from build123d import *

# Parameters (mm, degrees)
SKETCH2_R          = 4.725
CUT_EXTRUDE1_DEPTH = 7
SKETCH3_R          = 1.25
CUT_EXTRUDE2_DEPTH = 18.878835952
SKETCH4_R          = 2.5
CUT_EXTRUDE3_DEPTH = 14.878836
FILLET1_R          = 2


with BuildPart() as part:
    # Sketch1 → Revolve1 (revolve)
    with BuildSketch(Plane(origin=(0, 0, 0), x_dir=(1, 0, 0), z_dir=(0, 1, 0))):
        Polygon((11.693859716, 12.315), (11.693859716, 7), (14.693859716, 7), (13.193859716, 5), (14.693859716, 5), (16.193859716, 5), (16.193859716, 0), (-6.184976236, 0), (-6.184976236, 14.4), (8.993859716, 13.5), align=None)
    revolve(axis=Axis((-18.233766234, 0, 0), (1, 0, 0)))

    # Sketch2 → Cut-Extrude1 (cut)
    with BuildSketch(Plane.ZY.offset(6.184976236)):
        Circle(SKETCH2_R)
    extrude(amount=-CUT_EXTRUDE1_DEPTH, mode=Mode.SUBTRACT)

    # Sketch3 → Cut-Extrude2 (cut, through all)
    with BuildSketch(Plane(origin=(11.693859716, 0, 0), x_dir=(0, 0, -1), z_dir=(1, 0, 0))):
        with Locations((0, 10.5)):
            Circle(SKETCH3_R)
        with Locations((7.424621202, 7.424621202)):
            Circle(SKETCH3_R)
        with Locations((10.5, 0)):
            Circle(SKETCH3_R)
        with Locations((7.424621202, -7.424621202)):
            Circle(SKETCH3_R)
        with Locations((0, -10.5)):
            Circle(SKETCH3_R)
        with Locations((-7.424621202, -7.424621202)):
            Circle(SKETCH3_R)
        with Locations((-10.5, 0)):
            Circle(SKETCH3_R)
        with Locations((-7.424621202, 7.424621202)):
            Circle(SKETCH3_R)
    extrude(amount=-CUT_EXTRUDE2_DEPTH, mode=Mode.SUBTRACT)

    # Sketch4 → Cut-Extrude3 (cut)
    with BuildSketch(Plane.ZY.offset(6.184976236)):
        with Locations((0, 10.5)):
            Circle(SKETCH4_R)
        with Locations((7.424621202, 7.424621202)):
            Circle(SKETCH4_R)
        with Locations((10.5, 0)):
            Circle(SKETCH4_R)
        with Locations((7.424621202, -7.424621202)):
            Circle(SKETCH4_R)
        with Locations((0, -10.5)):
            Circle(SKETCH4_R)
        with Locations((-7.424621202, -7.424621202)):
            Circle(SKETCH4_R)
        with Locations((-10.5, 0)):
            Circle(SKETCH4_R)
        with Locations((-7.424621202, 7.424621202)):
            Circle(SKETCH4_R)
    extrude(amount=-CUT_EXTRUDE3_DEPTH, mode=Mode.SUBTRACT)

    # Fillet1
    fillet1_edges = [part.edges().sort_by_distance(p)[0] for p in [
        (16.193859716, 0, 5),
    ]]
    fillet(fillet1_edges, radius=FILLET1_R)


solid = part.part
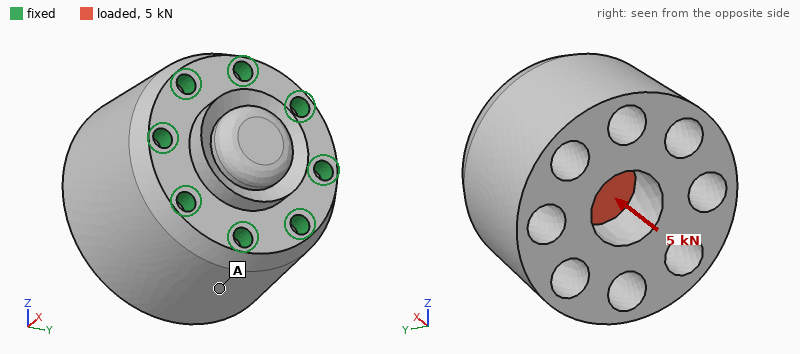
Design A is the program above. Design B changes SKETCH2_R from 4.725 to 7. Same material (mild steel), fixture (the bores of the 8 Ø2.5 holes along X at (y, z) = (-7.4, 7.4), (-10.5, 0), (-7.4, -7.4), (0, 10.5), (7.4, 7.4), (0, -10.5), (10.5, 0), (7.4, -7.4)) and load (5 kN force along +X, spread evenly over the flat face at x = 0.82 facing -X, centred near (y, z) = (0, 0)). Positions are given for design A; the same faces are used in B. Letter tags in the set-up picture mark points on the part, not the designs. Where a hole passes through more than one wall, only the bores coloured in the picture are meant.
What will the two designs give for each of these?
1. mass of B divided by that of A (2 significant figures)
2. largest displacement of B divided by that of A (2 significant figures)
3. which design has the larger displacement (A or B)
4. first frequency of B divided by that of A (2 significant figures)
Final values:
0.93
0.71
A
1.0
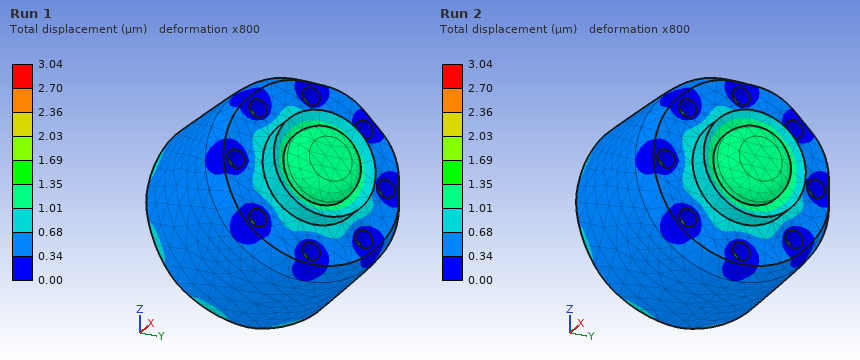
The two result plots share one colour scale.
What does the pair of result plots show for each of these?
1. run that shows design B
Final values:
Run 1
